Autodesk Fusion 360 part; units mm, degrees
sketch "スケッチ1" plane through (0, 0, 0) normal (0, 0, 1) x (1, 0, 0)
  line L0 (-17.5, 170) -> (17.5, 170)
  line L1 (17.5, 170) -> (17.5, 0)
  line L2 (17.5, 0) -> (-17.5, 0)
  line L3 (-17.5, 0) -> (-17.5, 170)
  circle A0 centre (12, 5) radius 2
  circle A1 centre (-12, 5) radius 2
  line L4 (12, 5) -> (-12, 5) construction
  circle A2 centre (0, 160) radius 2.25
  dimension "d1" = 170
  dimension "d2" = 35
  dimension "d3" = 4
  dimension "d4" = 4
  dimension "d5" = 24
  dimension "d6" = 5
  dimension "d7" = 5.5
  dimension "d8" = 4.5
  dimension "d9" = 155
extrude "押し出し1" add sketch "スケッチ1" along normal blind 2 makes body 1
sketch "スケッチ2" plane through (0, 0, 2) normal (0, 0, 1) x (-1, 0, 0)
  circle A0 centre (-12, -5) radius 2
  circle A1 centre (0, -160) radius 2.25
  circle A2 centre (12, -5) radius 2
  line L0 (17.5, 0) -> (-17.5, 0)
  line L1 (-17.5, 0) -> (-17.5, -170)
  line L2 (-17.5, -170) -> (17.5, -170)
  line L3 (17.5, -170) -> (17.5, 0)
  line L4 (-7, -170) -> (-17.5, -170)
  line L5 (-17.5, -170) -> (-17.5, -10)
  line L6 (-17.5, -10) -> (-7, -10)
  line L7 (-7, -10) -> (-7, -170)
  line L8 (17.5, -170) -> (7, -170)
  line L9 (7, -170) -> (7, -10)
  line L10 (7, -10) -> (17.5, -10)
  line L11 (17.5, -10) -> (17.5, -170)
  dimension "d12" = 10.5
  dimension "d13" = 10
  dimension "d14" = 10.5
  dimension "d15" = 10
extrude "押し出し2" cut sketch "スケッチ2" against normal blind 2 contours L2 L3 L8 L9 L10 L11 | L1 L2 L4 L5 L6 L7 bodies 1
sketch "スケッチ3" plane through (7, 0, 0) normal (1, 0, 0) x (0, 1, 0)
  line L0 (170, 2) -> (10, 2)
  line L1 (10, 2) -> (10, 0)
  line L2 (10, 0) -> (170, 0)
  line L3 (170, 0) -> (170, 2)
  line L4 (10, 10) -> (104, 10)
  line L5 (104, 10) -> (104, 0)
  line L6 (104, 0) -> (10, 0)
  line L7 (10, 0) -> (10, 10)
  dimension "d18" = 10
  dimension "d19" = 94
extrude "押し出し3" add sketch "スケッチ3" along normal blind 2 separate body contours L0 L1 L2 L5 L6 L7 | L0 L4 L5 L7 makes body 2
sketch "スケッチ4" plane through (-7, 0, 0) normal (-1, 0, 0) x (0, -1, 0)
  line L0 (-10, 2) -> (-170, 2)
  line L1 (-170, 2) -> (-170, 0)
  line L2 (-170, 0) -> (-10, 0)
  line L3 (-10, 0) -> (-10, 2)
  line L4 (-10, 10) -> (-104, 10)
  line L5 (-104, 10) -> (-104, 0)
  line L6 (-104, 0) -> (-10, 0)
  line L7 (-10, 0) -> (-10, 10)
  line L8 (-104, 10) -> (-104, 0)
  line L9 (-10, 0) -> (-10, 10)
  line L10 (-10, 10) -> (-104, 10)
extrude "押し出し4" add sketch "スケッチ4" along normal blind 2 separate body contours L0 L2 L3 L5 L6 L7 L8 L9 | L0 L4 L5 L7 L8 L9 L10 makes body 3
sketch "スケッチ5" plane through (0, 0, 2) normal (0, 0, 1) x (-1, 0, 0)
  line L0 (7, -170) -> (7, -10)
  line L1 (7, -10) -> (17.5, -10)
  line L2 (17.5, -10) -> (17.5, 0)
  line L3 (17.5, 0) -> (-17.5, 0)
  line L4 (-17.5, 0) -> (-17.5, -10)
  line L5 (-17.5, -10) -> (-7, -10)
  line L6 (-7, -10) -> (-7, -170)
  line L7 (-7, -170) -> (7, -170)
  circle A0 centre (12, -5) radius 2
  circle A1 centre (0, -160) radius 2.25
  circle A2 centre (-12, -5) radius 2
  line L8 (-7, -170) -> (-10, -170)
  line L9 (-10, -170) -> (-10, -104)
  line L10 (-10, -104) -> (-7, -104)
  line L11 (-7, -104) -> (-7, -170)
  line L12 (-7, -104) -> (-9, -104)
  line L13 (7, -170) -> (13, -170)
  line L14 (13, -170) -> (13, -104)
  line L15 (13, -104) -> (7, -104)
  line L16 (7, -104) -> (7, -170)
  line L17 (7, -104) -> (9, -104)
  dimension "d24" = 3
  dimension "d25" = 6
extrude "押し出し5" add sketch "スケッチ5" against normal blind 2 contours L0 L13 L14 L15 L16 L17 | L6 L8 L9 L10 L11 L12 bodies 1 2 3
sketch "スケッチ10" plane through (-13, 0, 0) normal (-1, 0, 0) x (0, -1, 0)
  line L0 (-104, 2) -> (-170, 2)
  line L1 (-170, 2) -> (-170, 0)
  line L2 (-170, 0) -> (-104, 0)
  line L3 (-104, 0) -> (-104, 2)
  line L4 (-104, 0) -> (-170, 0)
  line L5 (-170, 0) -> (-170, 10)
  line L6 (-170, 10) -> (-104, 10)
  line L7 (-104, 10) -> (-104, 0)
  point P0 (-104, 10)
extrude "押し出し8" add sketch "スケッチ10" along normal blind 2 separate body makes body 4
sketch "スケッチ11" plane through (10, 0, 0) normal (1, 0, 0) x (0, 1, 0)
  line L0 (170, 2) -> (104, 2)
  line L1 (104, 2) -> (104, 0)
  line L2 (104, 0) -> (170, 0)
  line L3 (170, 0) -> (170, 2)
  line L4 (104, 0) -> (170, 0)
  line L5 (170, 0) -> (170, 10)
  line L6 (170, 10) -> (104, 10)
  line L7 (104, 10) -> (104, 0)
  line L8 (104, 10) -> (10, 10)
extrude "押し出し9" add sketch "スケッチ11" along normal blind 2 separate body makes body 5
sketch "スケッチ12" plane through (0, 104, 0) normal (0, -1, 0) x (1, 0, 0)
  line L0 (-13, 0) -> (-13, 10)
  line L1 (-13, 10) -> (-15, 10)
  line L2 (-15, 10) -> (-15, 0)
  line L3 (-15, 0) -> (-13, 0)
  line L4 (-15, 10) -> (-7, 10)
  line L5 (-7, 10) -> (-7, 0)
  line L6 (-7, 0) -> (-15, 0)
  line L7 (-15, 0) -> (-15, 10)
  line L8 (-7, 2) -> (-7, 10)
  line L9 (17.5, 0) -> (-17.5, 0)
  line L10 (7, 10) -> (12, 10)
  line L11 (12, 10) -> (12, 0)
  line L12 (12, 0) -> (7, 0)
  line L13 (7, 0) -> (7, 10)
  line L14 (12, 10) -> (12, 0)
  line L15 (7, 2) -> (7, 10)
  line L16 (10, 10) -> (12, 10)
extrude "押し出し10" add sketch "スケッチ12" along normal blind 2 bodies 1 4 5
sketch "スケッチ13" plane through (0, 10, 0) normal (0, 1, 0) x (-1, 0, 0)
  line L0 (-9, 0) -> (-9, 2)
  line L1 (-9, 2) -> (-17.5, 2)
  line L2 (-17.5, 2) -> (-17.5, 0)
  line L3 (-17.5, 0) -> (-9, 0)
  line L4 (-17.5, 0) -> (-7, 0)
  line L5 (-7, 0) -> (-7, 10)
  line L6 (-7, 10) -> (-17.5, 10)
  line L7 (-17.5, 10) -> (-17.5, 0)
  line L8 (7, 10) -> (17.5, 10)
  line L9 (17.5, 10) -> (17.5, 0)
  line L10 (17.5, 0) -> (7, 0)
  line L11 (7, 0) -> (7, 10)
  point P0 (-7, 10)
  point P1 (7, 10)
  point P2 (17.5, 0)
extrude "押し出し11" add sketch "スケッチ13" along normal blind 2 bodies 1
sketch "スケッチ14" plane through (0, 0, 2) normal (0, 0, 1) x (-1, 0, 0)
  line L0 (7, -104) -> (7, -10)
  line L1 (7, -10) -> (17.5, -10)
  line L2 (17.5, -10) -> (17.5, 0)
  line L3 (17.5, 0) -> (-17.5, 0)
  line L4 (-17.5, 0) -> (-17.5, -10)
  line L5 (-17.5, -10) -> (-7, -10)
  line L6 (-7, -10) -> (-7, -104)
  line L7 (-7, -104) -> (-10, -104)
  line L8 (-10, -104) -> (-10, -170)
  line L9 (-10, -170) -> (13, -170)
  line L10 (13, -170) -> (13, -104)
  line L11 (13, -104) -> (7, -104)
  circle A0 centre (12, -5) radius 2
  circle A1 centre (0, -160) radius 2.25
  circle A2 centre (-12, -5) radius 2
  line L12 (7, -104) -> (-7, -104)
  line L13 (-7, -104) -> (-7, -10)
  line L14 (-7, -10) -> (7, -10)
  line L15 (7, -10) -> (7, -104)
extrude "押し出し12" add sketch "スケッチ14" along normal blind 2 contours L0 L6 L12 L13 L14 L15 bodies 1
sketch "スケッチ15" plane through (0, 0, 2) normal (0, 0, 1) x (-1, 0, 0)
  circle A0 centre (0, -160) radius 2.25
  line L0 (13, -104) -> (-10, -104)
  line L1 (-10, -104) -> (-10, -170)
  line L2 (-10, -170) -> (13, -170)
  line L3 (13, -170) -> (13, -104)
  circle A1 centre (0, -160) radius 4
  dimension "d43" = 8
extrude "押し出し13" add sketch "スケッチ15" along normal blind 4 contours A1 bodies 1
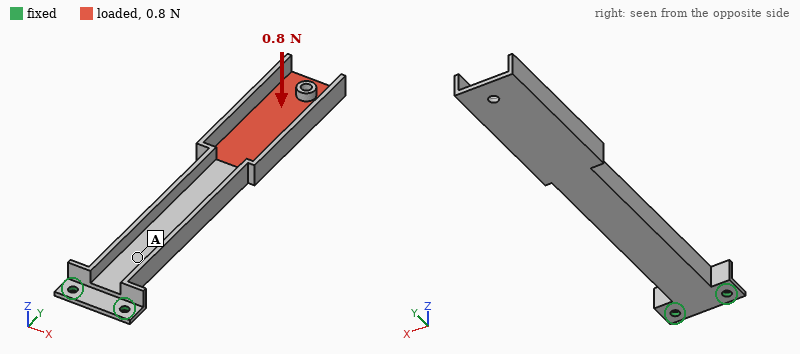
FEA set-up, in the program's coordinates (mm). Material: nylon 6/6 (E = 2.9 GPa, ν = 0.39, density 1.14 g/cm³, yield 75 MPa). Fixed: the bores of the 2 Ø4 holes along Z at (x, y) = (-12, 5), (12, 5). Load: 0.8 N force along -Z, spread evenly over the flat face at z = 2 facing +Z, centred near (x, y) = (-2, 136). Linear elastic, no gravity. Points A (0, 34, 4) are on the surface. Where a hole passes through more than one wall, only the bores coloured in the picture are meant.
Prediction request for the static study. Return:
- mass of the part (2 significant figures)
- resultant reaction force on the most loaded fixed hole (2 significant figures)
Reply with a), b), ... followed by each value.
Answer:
a) 18 g
b) 2.0 N
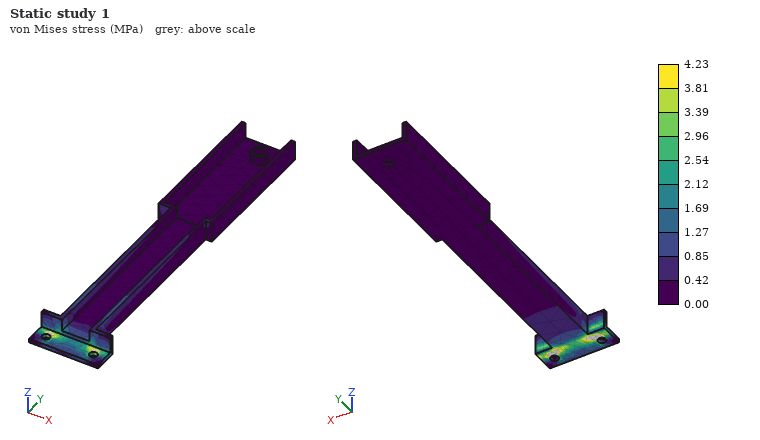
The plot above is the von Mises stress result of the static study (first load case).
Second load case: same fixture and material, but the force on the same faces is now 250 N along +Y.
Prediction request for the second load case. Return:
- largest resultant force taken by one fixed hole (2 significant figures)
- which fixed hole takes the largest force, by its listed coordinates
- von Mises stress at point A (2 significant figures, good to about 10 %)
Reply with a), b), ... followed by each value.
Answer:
a) 150 N
b) (-12, 5)
c) 2.3 MPa
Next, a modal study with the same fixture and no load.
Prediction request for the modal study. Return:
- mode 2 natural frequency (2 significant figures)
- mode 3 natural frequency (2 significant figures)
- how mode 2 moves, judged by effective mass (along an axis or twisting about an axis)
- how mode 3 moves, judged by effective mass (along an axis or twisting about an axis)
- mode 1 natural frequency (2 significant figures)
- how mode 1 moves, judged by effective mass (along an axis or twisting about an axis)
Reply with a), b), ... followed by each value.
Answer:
a) 170 Hz
b) 300 Hz
c) along X
d) twisting about Y
e) 39 Hz
f) along Z
